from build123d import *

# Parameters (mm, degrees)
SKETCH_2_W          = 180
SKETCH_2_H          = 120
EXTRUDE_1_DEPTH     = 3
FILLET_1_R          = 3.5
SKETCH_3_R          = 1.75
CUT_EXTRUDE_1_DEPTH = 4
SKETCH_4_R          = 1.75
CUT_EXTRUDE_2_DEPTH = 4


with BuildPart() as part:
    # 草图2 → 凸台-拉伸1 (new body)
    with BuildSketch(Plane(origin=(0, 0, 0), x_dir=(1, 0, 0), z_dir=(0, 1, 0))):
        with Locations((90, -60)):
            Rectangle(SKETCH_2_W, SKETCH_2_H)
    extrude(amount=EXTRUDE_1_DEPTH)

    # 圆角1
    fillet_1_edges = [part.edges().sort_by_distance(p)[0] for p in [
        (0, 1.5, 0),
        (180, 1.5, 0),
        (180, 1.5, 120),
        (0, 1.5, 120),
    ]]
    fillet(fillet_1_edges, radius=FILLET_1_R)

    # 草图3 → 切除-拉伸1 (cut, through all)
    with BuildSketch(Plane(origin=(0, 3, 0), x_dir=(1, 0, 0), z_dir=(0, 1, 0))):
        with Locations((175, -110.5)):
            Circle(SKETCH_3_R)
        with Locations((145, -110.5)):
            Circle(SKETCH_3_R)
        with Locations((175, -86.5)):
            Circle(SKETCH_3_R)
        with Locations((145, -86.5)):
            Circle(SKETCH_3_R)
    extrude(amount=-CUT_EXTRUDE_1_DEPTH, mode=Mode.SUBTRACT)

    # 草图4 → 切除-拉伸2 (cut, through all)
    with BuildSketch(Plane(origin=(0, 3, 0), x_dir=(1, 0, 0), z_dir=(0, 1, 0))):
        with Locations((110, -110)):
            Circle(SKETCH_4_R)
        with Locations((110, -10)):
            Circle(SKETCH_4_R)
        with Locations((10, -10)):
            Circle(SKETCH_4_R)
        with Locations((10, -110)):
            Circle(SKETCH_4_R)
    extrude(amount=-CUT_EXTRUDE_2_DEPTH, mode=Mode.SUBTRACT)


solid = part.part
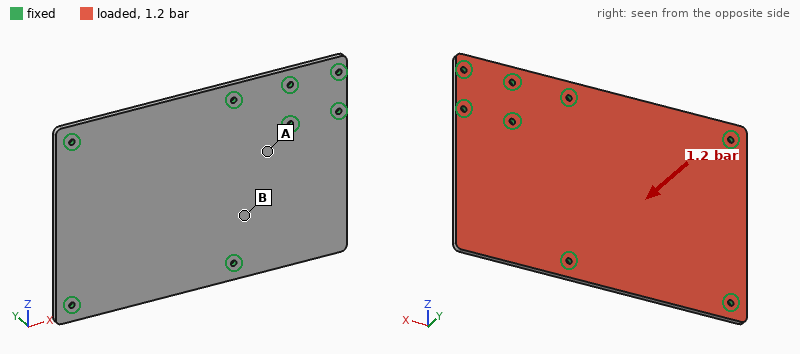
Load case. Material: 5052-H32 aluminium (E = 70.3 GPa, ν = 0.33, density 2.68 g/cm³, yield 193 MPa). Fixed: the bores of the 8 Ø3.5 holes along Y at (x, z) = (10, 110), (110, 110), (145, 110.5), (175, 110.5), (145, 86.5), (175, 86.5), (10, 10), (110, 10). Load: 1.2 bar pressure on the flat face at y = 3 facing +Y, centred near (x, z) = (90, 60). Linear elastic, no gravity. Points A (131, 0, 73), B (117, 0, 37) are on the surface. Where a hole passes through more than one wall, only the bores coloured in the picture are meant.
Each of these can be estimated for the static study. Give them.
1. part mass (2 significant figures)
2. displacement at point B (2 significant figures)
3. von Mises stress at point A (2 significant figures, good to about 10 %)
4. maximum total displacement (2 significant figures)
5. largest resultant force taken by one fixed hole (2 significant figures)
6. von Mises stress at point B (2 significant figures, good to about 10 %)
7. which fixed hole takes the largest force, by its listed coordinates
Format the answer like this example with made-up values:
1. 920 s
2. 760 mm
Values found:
1. 170 g
2. 0.18 mm
3. 23 MPa
4. 0.95 mm
5. 700 N
6. 57 MPa
7. (110, 10)
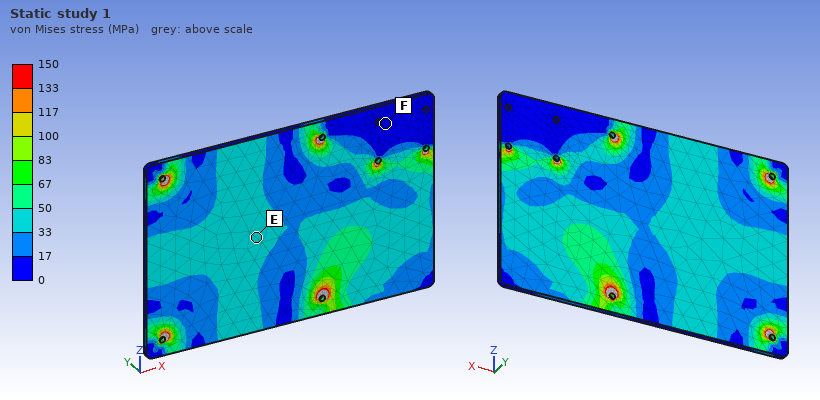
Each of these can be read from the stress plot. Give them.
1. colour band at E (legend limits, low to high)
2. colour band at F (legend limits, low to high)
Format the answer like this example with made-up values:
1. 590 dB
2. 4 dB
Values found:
1. 33 to 50 MPa
2. 0 to 17 MPa
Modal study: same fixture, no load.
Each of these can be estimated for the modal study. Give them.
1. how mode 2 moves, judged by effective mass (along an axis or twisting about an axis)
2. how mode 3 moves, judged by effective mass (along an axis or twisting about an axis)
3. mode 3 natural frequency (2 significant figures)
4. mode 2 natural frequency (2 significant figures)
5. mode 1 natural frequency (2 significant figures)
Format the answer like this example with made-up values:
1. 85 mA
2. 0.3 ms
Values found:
1. along Y
2. twisting about X
3. 1700 Hz
4. 1000 Hz
5. 810 Hz
